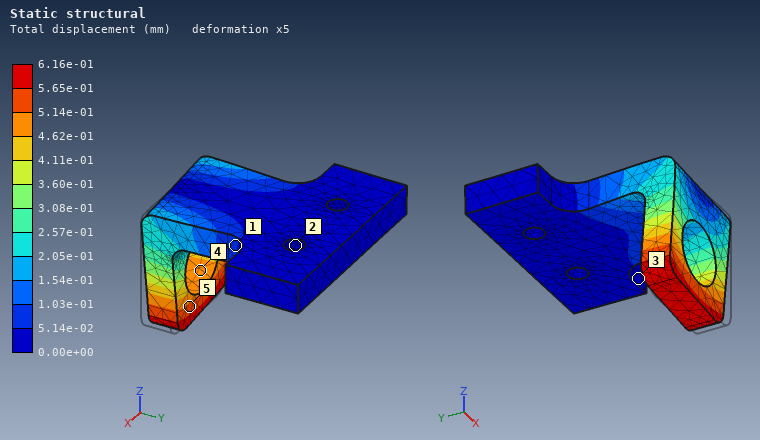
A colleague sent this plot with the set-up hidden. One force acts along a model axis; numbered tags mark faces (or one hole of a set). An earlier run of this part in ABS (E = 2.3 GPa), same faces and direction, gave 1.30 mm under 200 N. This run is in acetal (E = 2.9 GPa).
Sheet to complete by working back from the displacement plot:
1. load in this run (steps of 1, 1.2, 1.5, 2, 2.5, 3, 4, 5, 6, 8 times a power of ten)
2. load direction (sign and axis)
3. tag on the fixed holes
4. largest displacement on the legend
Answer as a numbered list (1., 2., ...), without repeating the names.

1. 120 N
2. -X
3. 2
4. 6.16e-01 mm
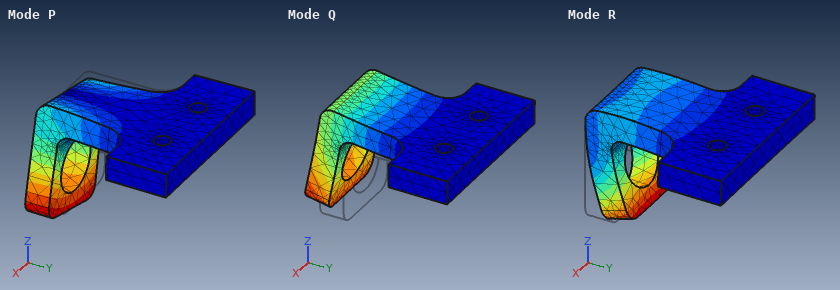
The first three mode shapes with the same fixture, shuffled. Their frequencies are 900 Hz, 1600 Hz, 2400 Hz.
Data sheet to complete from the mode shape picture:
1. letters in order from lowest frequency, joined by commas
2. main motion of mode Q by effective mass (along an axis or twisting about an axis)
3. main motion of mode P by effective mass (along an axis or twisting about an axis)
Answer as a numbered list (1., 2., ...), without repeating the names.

1. Q, P, R
2. along Z
3. along X
